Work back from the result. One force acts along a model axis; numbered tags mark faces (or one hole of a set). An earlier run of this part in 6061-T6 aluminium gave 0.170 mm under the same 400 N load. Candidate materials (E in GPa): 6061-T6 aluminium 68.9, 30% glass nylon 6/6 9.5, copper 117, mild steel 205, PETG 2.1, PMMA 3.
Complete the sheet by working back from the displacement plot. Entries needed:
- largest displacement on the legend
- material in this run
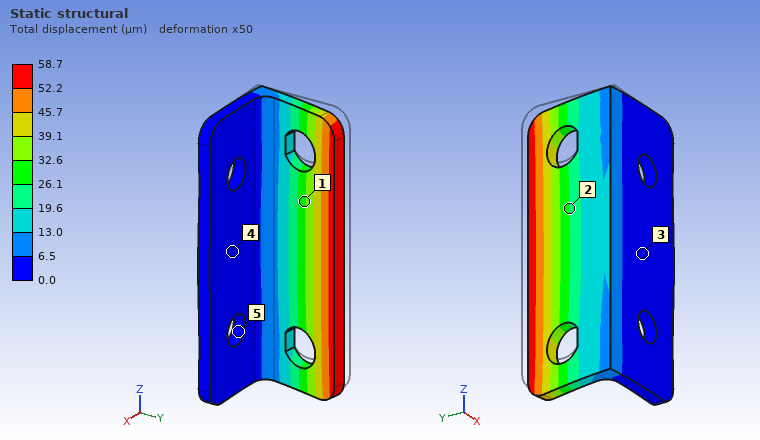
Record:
58.7 µm
mild steel
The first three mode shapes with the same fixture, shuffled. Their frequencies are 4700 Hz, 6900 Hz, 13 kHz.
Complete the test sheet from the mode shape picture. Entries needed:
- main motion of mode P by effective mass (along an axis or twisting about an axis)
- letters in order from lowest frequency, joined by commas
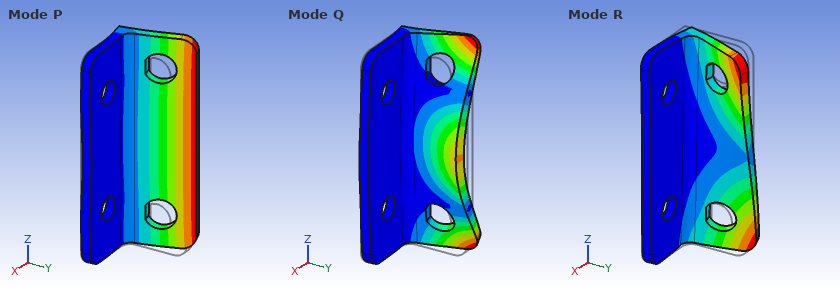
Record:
along X
P, R, Q
